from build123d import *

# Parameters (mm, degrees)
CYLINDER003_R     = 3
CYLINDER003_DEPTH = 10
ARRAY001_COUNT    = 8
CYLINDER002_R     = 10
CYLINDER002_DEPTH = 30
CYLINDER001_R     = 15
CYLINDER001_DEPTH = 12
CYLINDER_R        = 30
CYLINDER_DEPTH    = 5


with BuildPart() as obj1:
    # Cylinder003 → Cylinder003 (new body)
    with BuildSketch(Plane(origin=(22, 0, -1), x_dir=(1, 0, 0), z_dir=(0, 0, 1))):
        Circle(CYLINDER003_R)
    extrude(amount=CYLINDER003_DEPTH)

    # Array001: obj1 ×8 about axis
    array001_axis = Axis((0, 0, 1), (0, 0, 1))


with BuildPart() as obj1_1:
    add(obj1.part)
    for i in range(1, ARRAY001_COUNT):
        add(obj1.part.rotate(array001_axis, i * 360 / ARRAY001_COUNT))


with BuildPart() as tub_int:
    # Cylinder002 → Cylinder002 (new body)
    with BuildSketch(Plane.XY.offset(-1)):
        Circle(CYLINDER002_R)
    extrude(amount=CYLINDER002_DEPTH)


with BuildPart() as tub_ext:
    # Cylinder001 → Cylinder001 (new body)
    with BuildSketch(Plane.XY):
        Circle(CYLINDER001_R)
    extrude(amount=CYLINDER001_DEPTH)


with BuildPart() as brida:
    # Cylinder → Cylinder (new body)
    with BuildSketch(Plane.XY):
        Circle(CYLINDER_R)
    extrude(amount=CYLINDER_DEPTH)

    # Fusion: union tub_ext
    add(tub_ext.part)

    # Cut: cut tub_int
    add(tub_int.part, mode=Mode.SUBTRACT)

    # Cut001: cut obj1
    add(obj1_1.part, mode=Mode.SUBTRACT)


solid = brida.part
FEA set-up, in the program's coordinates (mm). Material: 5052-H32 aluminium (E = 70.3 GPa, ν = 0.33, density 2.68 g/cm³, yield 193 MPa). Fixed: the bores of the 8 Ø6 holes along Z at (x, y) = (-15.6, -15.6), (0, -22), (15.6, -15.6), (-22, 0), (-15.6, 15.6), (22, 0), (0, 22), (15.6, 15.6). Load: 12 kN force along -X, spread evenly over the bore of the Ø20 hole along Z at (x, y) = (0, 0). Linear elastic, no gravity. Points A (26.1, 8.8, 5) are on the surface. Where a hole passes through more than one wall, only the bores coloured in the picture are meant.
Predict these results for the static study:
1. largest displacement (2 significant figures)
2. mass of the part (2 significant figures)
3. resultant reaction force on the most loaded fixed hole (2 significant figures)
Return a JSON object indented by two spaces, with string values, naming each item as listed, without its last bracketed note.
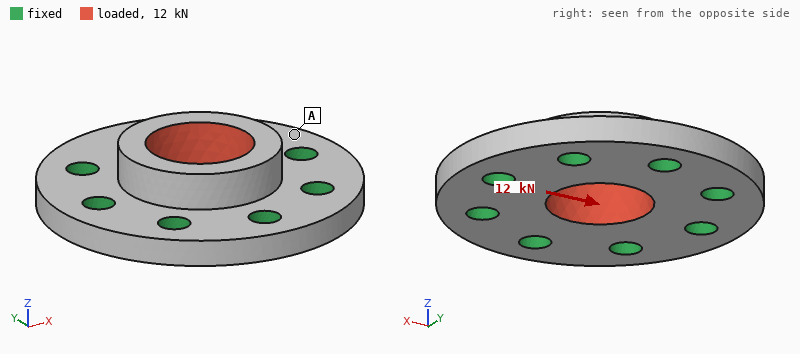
{
  "largest displacement": "16 µm",
  "mass of the part": "38 g",
  "resultant reaction force on the most loaded fixed hole": "2.3 kN"
}
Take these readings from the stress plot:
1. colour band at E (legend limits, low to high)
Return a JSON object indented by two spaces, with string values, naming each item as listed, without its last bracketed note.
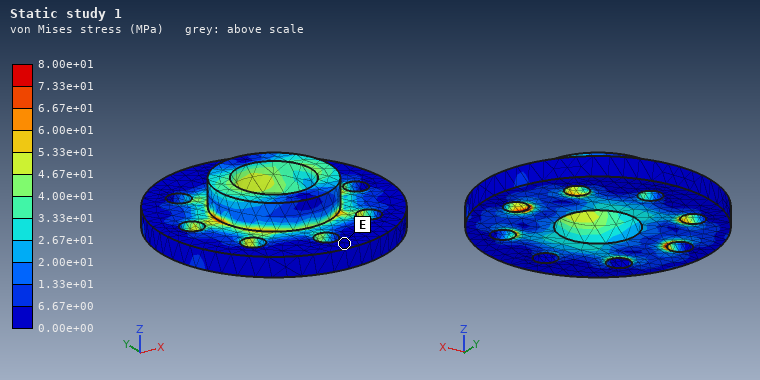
{
  "colour band at E": "0.00e+00 to 6.67e+00 MPa"
}
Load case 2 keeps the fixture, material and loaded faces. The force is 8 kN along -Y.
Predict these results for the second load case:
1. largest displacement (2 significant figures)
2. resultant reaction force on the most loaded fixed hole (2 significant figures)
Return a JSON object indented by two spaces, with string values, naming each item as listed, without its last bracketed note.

{
  "largest displacement": "11 µm",
  "resultant reaction force on the most loaded fixed hole": "1.5 kN"
}
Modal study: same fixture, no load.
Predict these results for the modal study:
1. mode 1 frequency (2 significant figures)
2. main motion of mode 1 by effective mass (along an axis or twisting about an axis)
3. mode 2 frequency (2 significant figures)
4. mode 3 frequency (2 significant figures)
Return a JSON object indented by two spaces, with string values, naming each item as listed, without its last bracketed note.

{
  "mode 1 frequency": "36 kHz",
  "main motion of mode 1 by effective mass": "along Z",
  "mode 2 frequency": "45 kHz",
  "mode 3 frequency": "45 kHz"
}
